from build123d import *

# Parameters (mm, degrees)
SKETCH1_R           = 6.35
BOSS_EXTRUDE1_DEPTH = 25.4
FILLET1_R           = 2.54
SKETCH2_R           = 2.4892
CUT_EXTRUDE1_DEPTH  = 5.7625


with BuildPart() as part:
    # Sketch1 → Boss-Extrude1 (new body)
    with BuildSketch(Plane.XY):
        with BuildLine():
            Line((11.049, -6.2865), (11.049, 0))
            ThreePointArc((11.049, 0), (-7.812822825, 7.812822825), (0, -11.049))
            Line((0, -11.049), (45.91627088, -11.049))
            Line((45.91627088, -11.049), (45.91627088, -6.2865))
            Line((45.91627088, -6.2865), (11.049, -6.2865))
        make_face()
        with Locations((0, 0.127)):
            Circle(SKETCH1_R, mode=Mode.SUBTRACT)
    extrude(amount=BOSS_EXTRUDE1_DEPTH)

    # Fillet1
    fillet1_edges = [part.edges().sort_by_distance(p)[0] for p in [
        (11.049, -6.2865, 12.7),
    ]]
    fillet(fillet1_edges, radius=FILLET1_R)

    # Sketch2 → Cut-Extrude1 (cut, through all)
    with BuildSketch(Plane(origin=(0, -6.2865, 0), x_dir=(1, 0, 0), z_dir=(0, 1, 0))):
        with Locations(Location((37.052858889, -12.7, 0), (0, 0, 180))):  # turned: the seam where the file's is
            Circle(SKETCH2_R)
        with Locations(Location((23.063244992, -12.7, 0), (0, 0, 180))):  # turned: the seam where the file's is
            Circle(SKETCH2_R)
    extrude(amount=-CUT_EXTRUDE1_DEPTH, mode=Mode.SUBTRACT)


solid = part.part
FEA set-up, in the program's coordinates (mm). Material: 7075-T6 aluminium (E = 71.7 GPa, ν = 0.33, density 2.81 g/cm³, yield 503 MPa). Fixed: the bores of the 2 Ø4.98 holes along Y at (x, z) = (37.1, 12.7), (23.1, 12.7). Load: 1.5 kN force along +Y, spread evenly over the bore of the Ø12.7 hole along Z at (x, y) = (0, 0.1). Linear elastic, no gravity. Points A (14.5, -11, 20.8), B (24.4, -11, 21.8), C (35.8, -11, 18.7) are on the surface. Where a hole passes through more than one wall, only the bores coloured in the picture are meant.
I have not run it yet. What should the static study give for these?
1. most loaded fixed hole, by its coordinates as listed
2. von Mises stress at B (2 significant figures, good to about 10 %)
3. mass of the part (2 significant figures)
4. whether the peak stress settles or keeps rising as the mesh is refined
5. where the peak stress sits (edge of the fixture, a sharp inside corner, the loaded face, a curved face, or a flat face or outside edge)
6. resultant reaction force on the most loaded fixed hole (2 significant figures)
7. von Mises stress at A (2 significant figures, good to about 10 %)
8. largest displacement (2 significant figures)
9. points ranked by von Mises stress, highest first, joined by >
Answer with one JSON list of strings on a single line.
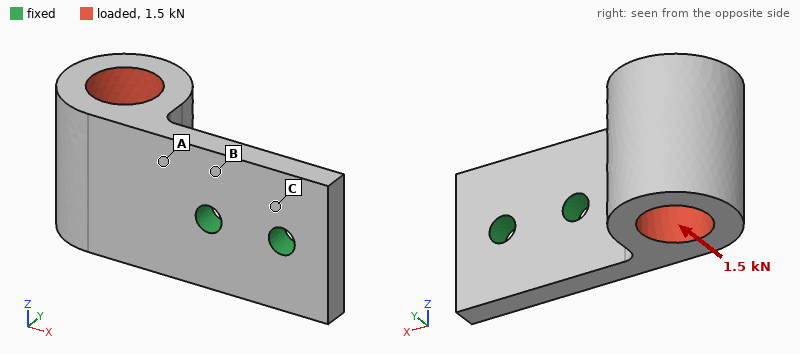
["(23.1, 12.7)", "130 MPa", "32 g", "keeps rising", "edge of the fixture", "2.2 kN", "200 MPa", "0.60 mm", "A > B > C"]
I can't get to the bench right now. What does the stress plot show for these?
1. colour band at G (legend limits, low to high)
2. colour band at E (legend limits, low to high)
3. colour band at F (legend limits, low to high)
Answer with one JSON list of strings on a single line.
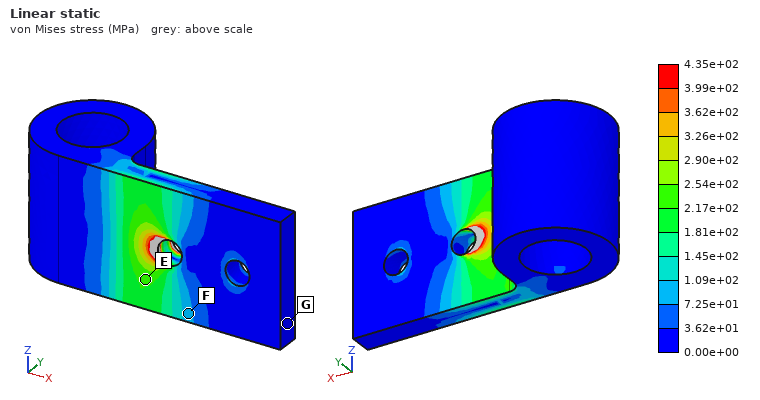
["0.00e+00 to 3.62e+01 MPa", "2.17e+02 to 2.54e+02 MPa", "7.25e+01 to 1.09e+02 MPa"]
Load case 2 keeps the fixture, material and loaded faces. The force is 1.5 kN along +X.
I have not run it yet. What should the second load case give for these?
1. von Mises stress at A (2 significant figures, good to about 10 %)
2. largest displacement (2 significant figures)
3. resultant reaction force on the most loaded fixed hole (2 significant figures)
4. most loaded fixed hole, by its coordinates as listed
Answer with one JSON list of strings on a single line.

["110 MPa", "0.31 mm", "1.2 kN", "(23.1, 12.7)"]
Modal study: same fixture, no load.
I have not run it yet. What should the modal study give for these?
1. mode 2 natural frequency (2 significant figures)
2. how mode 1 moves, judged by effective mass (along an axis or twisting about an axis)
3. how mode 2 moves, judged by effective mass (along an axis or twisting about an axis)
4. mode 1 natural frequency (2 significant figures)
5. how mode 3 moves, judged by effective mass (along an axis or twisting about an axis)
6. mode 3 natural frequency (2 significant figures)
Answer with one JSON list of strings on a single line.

["4000 Hz", "along Y", "along Z", "2000 Hz", "along Z", "8000 Hz"]
